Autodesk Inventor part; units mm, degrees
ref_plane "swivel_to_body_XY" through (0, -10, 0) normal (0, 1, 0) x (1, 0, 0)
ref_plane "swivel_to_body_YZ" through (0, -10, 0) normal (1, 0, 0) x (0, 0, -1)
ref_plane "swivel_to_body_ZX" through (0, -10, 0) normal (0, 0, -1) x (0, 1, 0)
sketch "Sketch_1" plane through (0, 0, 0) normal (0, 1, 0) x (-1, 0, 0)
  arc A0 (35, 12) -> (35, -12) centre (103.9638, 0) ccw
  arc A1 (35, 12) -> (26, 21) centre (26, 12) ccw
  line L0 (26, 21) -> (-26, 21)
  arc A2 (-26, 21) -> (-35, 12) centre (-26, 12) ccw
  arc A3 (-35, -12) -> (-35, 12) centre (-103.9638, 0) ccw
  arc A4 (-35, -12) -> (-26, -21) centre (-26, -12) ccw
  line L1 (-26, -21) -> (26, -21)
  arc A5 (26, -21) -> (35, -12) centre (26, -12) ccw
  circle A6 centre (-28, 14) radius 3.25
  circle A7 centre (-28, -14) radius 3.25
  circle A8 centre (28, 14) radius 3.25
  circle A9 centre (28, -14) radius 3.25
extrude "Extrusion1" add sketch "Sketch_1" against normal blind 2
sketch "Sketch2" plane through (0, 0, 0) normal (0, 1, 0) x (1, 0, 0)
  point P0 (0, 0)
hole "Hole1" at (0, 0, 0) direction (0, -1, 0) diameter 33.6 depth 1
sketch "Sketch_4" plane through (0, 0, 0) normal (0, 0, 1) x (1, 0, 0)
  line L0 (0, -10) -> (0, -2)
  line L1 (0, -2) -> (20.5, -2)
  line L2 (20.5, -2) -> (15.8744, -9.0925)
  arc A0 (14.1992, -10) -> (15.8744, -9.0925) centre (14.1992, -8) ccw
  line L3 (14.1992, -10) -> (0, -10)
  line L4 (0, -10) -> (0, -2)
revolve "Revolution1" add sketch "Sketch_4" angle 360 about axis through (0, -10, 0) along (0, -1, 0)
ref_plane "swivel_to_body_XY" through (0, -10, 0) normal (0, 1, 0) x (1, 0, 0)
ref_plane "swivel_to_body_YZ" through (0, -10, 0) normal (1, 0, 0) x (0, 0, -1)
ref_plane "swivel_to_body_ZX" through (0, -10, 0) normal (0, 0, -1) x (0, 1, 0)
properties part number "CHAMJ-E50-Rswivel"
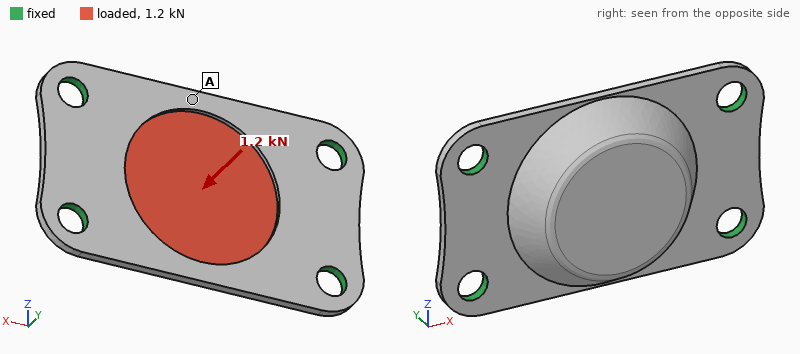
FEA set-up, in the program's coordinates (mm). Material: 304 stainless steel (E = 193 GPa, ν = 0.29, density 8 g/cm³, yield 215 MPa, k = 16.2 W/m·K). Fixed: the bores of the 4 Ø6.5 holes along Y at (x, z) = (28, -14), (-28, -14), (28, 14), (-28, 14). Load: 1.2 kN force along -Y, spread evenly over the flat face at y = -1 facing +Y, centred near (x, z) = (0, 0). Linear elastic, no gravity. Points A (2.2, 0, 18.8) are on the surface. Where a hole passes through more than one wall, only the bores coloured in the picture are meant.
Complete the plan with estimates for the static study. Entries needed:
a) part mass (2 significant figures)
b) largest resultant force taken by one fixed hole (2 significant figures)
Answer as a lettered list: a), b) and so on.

a) 100 g
b) 490 N
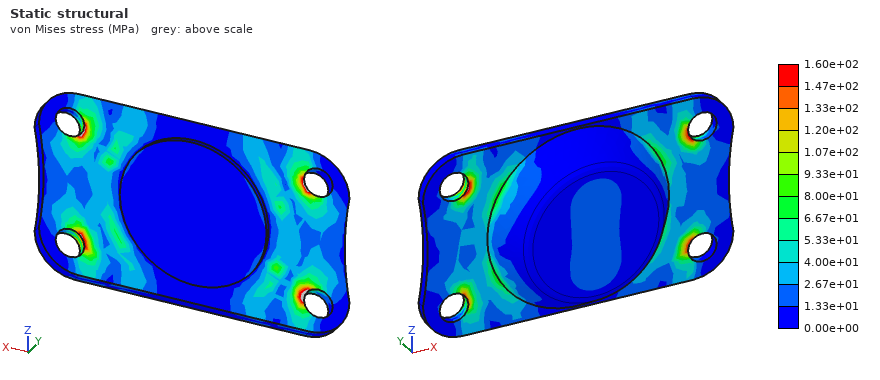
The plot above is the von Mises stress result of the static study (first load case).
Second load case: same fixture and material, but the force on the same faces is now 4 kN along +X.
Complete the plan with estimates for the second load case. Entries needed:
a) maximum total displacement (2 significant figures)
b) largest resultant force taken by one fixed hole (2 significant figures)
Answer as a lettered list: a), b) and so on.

a) 3.3 µm
b) 1.0 kN
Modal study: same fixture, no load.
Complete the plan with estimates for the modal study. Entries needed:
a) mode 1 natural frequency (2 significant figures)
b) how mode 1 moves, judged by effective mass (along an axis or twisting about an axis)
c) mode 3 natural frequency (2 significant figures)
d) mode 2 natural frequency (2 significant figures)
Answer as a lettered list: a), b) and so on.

a) 4900 Hz
b) along Y
c) 10 kHz
d) 5500 Hz
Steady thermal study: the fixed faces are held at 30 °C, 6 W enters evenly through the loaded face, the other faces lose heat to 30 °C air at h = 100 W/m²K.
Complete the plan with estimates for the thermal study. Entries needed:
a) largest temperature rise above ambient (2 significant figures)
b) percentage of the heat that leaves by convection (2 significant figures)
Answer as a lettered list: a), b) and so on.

a) 16 K
b) 69 %
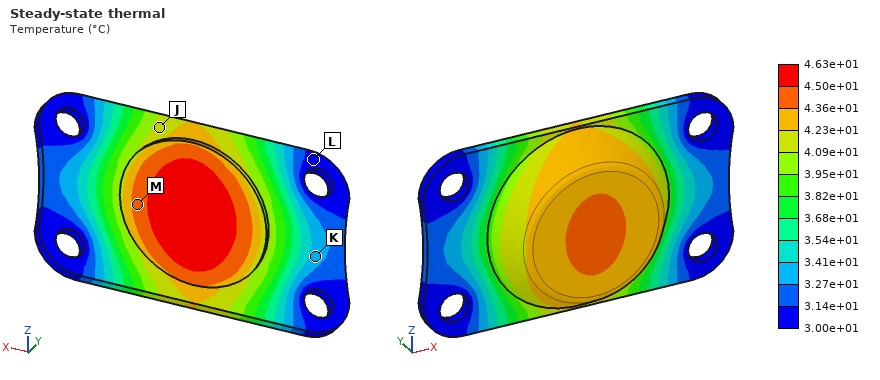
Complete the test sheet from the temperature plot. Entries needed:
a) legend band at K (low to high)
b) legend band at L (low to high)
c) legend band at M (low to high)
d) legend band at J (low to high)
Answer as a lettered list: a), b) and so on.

a) 3.27e+01 to 3.41e+01 °C
b) 3.00e+01 to 3.14e+01 °C
c) 4.36e+01 to 4.50e+01 °C
d) 4.09e+01 to 4.23e+01 °C
